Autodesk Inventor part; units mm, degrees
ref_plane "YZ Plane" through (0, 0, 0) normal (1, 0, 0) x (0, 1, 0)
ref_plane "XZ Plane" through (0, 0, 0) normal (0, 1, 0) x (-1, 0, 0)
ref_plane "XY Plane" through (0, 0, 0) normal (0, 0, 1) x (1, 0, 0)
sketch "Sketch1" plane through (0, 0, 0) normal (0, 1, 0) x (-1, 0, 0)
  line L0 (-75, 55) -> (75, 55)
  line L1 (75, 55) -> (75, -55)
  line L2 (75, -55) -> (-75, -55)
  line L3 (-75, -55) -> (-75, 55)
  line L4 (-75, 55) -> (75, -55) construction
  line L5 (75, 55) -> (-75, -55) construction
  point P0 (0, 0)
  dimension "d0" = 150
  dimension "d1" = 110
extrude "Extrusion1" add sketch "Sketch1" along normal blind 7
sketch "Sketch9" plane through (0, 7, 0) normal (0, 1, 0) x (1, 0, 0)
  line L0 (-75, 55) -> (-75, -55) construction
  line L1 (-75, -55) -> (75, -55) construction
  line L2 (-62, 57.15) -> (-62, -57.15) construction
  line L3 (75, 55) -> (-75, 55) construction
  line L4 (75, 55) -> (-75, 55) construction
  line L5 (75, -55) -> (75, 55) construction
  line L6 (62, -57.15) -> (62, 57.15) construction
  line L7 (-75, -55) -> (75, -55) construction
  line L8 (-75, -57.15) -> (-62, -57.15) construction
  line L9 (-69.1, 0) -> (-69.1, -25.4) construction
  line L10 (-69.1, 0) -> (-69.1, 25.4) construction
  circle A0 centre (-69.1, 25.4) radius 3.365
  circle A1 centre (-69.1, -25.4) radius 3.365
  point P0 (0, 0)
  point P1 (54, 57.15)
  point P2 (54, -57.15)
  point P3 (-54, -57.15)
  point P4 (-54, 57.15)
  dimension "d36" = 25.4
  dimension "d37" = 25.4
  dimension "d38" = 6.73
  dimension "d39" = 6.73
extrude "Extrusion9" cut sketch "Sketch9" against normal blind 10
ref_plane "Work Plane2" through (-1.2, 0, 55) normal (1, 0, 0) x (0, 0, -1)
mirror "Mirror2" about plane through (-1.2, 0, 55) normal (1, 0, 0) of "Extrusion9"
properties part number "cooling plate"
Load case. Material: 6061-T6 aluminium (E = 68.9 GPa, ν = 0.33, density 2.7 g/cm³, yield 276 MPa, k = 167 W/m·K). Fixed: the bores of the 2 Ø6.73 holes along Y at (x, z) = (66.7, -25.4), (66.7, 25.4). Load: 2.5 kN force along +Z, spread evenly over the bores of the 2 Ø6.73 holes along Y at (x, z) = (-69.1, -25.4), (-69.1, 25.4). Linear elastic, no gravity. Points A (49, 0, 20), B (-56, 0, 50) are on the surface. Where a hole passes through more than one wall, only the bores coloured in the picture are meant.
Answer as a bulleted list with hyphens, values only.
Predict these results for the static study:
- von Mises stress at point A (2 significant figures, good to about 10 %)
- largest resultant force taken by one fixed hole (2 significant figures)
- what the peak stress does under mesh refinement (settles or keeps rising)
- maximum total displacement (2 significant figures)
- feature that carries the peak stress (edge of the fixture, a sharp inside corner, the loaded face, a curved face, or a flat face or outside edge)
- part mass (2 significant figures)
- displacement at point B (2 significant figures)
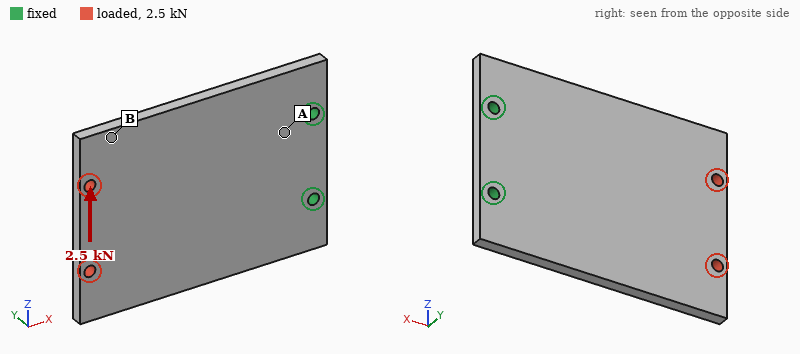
- 27 MPa
- 6.2 kN
- keeps rising
- 0.13 mm
- edge of the fixture
- 310 g
- 0.11 mm
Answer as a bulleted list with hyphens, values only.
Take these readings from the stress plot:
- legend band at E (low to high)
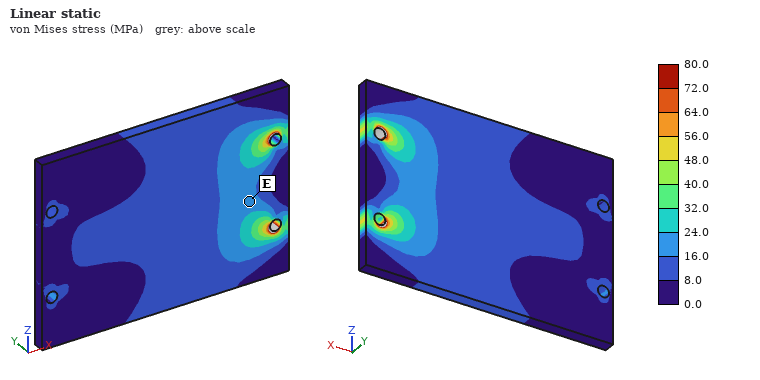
- 16.0 to 24.0 MPa
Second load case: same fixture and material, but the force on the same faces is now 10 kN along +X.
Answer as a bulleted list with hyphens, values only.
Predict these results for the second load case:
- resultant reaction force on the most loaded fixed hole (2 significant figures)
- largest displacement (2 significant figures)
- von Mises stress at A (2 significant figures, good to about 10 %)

- 5.0 kN
- 46 µm
- 22 MPa
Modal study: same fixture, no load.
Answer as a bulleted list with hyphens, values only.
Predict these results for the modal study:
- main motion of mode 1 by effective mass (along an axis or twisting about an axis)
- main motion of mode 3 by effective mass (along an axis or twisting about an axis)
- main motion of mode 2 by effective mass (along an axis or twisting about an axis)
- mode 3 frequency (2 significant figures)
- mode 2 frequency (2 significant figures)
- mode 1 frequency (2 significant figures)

- along Y
- along Y
- twisting about X
- 1700 Hz
- 790 Hz
- 270 Hz
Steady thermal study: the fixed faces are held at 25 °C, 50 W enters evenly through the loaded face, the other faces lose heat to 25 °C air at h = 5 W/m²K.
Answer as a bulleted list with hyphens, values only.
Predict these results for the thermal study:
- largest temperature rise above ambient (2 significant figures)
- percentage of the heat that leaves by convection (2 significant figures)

- 60 K
- 9.9 %
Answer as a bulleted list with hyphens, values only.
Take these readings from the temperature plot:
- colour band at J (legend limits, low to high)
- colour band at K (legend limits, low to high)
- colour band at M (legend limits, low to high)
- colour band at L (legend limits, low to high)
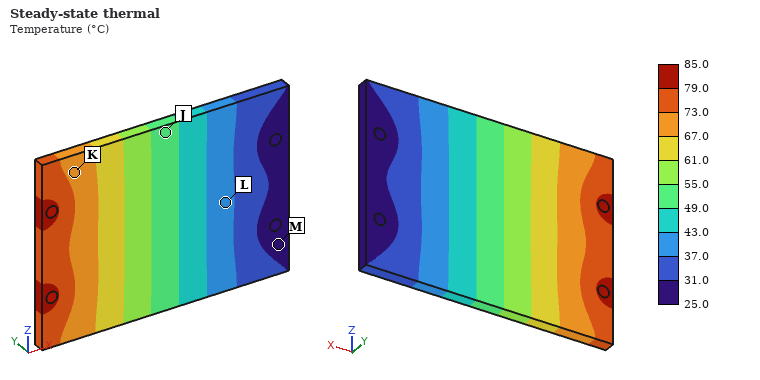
- 49.0 to 55.0 °C
- 67.0 to 73.0 °C
- 25.0 to 31.0 °C
- 37.0 to 43.0 °C
